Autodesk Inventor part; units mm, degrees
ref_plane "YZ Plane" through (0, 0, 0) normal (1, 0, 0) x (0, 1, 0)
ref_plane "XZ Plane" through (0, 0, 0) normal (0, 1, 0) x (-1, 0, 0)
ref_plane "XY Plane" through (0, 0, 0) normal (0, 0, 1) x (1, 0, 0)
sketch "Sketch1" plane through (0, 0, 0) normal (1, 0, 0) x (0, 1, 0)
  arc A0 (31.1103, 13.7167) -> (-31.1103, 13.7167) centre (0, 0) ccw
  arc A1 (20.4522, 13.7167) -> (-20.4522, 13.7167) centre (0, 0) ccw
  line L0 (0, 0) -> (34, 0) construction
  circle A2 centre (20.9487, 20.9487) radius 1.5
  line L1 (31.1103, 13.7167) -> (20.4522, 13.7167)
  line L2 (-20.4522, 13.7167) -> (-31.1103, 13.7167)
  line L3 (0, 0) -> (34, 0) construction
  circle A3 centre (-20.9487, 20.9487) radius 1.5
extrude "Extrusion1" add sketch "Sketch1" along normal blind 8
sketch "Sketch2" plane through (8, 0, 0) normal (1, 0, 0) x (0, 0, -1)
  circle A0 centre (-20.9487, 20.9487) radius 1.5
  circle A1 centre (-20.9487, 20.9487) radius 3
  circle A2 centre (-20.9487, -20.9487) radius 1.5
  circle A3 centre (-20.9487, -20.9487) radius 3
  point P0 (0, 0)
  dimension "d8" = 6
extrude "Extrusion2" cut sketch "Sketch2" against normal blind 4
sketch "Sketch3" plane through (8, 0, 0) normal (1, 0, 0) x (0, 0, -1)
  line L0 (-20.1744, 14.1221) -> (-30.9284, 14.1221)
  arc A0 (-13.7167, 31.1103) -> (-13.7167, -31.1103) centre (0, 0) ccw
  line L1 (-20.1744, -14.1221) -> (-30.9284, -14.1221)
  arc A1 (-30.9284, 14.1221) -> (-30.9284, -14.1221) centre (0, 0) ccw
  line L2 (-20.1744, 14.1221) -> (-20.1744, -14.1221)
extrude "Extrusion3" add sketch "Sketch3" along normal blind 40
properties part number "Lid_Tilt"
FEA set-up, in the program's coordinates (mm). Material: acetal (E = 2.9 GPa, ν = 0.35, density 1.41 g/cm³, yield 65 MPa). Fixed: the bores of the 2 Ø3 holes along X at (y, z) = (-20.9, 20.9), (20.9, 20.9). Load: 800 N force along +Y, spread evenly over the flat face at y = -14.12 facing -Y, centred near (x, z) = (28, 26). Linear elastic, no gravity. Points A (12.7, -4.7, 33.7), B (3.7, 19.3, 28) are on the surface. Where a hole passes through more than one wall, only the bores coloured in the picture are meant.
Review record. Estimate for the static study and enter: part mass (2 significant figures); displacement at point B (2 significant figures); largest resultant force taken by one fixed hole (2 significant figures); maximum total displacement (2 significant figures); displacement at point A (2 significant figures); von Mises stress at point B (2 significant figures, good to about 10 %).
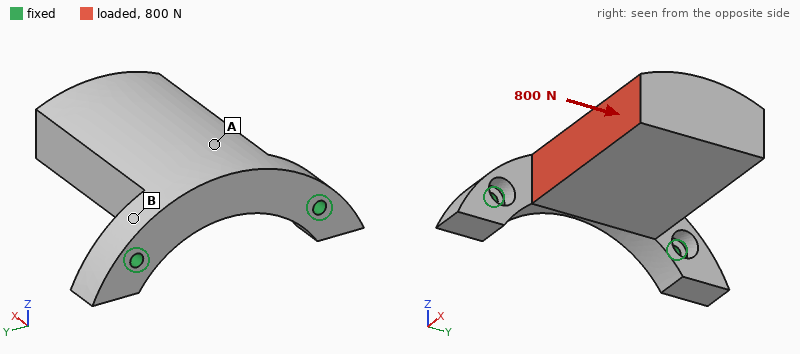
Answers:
27 g
0.10 mm
670 N
0.62 mm
0.099 mm
12 MPa
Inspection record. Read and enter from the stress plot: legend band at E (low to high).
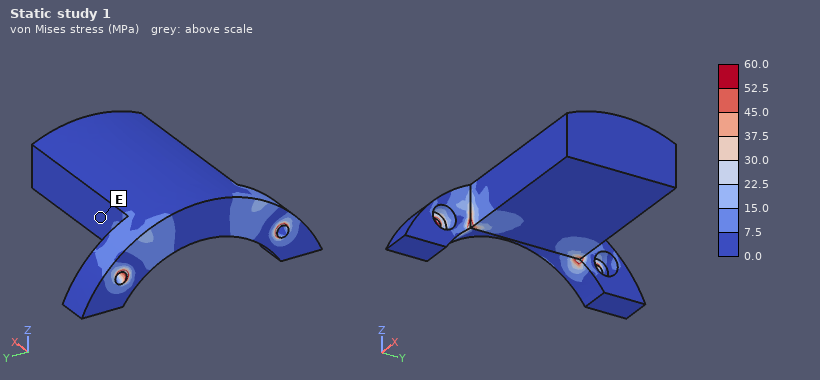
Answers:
0.0 to 7.5 MPa
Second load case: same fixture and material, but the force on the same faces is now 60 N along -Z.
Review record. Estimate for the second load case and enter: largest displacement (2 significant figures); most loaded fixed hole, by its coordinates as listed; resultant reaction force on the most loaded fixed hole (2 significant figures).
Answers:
0.74 mm
(-20.9, 20.9)
57 N
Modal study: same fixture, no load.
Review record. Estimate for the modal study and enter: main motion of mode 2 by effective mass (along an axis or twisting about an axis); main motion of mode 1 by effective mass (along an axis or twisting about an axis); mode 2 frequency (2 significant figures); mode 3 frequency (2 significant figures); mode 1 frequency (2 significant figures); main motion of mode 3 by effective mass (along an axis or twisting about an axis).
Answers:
along Y
along Z
1600 Hz
2400 Hz
390 Hz
along X
